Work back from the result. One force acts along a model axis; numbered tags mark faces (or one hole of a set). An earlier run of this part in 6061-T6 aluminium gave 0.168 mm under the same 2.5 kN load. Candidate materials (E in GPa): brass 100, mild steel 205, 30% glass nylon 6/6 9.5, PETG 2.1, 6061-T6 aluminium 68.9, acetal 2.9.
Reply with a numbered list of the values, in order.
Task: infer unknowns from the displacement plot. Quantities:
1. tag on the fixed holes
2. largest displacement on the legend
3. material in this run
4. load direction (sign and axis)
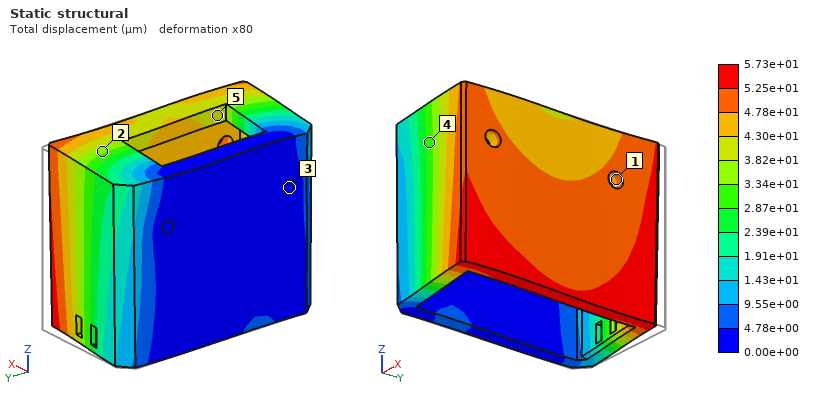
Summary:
1. 3
2. 5.73e+01 µm
3. mild steel
4. -Y
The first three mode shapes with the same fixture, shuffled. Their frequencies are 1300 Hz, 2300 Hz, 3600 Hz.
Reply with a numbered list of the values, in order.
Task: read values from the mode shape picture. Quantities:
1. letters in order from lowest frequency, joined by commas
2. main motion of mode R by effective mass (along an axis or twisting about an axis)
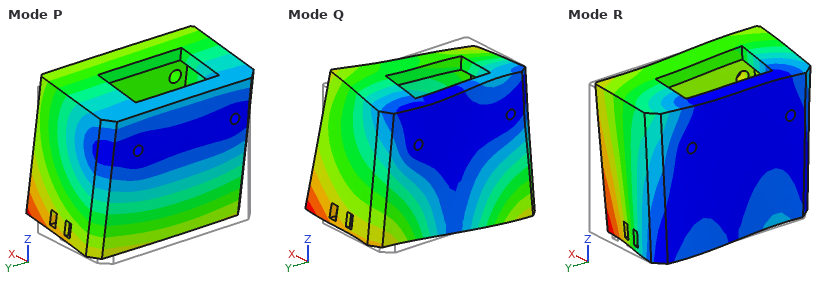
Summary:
1. P, R, Q
2. along Y
